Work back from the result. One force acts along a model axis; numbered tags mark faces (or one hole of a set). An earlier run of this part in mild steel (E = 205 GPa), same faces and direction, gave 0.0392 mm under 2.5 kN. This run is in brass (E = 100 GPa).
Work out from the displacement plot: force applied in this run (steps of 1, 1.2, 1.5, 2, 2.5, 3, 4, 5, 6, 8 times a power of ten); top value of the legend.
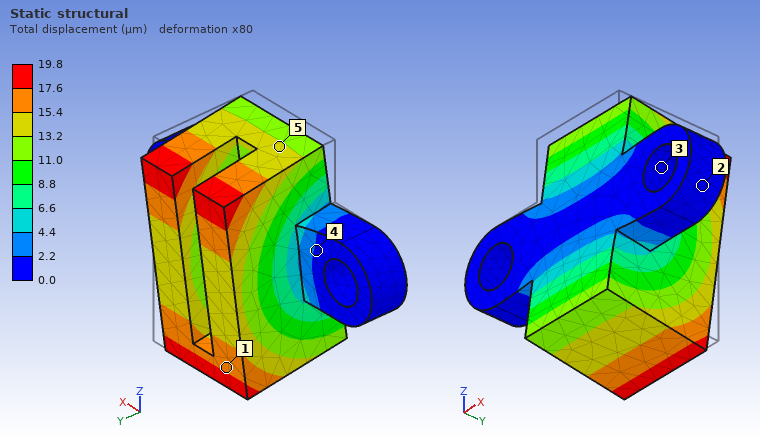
600 N
19.8 µm
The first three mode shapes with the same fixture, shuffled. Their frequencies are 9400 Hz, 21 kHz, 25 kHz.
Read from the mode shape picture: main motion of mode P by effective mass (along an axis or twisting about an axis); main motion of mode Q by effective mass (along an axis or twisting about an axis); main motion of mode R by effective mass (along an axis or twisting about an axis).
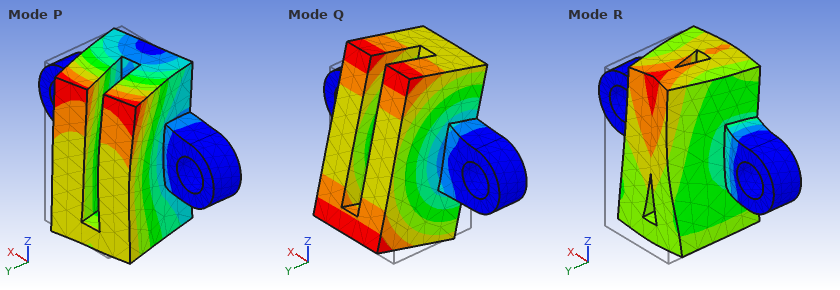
along X
along Z
along Y
